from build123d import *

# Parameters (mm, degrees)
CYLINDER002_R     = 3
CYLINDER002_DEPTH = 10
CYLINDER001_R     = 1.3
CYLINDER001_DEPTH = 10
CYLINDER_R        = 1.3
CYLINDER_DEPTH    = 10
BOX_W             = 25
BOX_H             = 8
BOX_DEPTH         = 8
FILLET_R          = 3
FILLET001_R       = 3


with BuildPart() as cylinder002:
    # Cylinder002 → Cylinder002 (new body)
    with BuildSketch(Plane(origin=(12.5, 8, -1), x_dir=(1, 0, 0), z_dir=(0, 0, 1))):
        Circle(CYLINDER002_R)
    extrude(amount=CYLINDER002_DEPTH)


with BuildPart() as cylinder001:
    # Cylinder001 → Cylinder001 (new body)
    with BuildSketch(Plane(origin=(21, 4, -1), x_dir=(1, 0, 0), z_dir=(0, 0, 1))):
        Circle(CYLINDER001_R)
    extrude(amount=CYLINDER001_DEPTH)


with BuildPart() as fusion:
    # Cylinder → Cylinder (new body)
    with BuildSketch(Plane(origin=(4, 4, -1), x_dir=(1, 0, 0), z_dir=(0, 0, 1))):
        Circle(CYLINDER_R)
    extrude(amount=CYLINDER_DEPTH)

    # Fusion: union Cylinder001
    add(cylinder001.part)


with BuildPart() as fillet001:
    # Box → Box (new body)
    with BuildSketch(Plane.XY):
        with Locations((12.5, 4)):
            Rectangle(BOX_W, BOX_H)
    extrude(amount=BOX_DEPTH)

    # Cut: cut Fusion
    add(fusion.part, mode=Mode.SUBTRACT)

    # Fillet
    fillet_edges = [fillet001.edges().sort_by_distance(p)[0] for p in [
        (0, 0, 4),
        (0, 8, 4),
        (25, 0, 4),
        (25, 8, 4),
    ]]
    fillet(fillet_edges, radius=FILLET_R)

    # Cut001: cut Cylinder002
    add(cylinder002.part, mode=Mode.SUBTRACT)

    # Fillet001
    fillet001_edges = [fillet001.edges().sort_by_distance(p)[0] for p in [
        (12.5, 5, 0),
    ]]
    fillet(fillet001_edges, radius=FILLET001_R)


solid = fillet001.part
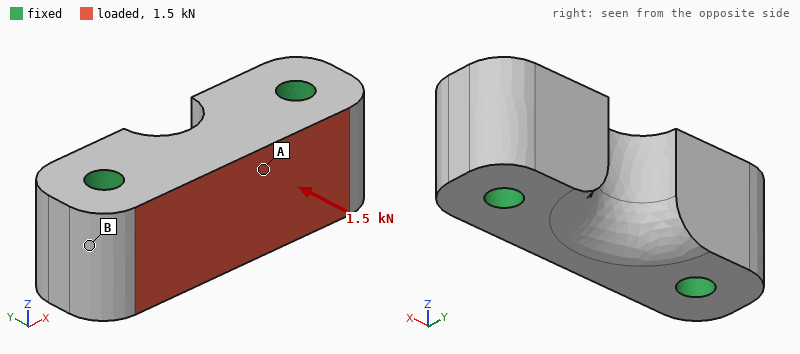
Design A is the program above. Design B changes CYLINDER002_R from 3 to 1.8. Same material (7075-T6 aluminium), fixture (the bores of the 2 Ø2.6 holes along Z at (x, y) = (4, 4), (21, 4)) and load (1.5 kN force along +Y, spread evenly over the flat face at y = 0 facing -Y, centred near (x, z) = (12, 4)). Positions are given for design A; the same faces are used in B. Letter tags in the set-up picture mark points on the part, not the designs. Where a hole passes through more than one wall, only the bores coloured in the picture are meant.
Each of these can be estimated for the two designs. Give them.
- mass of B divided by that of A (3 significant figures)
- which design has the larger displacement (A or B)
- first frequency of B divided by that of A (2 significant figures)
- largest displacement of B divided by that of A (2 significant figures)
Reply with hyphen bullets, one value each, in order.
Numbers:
- 1.06
- A
- 0.97
- 0.91
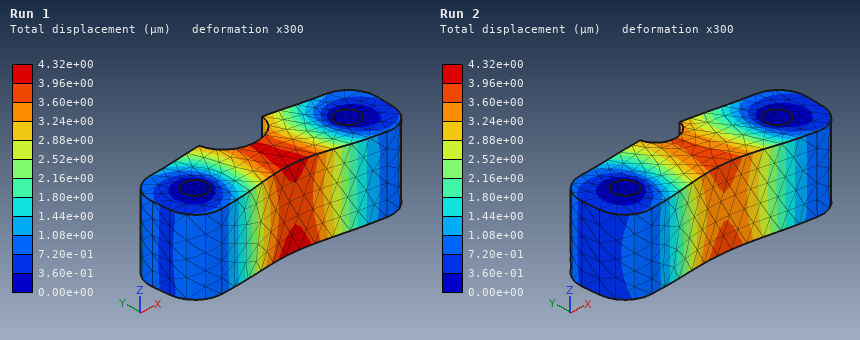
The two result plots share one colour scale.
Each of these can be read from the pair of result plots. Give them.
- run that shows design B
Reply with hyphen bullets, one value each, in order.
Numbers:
- Run 2
